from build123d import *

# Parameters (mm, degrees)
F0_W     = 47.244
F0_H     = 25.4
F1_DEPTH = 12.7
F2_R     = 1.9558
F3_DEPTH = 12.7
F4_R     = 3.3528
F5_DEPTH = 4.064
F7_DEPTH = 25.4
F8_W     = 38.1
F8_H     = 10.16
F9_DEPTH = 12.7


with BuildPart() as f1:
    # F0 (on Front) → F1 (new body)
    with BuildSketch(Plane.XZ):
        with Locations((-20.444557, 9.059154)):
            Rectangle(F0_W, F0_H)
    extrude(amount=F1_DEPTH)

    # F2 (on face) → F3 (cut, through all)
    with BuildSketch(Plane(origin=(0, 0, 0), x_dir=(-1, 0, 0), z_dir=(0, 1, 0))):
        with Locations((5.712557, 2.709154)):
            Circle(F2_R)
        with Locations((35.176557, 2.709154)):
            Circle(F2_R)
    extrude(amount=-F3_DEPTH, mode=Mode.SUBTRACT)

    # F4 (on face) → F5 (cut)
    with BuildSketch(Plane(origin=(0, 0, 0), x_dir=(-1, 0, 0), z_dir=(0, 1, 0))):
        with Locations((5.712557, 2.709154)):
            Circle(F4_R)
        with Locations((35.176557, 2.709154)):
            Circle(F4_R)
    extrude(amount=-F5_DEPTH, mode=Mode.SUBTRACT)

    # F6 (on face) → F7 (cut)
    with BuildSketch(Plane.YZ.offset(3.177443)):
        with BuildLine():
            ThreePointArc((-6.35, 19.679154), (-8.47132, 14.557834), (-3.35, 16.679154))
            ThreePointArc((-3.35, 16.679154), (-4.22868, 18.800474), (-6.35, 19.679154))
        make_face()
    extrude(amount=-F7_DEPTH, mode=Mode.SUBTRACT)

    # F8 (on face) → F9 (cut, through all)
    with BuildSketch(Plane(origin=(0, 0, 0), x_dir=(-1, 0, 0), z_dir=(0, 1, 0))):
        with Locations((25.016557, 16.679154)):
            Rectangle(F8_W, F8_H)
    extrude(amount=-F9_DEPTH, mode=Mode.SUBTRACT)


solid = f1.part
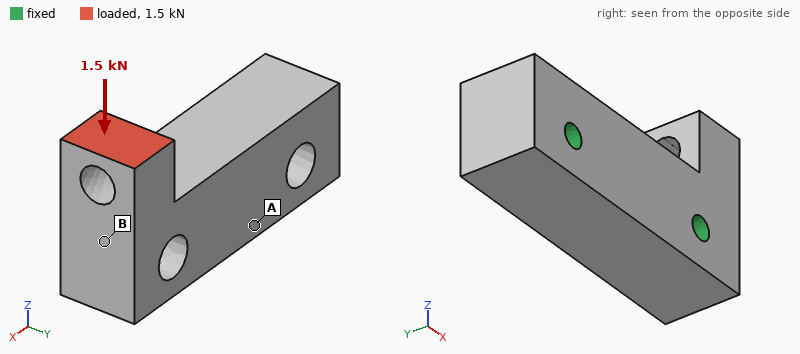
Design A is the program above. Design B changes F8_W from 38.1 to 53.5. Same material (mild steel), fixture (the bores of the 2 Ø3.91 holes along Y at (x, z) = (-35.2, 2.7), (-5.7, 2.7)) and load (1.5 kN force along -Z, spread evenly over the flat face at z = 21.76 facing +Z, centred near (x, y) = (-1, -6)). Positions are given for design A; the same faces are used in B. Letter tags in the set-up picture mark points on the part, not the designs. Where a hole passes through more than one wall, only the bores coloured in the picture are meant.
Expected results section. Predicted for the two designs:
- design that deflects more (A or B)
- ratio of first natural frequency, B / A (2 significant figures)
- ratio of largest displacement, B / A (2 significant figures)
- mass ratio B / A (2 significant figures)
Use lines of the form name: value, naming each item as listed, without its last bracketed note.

design that deflects more: B
ratio of first natural frequency, B / A: 0.50
ratio of largest displacement, B / A: 4.3
mass ratio B / A: 0.92
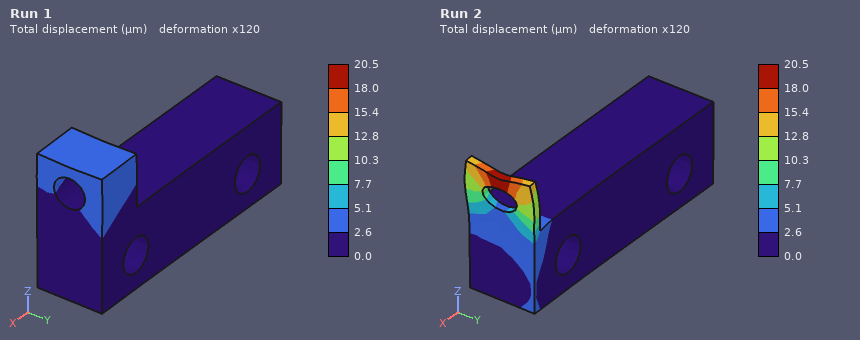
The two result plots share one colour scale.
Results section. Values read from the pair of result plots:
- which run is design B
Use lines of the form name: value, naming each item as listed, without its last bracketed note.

which run is design B: Run 2
